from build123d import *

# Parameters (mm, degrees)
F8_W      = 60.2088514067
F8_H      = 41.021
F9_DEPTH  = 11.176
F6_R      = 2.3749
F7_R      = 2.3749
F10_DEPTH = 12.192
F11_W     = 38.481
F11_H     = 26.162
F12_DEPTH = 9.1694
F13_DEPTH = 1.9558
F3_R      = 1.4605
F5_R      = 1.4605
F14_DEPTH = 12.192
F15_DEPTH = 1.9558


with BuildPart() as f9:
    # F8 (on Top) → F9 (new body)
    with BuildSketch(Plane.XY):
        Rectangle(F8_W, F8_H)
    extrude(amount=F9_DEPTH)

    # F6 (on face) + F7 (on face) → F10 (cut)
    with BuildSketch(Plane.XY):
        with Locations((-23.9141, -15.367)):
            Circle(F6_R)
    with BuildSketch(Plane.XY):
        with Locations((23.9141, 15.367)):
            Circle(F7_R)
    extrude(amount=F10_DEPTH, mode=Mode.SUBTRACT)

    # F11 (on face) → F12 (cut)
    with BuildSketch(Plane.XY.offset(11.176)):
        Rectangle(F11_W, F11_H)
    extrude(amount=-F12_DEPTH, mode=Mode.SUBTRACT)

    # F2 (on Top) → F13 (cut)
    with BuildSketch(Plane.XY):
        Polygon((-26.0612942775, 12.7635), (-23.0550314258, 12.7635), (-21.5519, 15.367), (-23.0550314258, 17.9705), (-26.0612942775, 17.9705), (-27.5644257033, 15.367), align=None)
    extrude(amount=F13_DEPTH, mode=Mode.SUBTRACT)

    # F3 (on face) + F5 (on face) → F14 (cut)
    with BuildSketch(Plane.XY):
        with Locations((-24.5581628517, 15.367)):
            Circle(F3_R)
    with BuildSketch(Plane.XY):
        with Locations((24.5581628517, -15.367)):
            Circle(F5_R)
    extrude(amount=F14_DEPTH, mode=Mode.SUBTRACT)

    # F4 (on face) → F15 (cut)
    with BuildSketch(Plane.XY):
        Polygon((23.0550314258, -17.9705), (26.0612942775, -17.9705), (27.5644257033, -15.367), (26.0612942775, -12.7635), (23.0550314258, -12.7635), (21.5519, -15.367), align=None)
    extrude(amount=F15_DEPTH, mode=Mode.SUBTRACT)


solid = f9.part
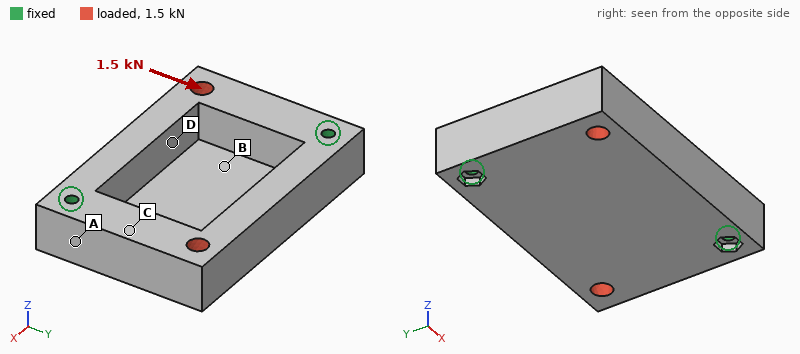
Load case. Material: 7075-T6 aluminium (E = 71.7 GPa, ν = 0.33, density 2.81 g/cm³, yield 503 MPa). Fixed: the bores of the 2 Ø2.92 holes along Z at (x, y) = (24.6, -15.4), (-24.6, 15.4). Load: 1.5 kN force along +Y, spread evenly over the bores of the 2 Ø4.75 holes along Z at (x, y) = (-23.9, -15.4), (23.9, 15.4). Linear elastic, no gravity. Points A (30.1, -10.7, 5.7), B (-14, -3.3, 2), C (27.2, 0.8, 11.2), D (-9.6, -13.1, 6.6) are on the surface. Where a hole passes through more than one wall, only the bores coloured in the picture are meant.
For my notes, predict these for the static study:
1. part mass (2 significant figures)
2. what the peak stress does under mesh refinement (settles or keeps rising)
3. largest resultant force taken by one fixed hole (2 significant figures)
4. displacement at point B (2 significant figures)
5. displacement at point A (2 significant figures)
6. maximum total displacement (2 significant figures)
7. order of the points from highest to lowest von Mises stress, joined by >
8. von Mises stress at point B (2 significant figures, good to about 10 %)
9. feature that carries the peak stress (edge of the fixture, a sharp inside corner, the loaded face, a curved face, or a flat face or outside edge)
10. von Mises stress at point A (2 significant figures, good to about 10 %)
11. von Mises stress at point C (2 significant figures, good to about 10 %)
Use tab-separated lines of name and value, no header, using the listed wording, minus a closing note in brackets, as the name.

part mass	50 g
what the peak stress does under mesh refinement	keeps rising
largest resultant force taken by one fixed hole	750 N
displacement at point B	1.8 µm
displacement at point A	0.65 µm
maximum total displacement	3.6 µm
order of the points from highest to lowest von Mises stress, joined by >	C > A > B > D
von Mises stress at point B	2.9 MPa
feature that carries the peak stress	edge of the fixture
von Mises stress at point A	4.9 MPa
von Mises stress at point C	6.7 MPa
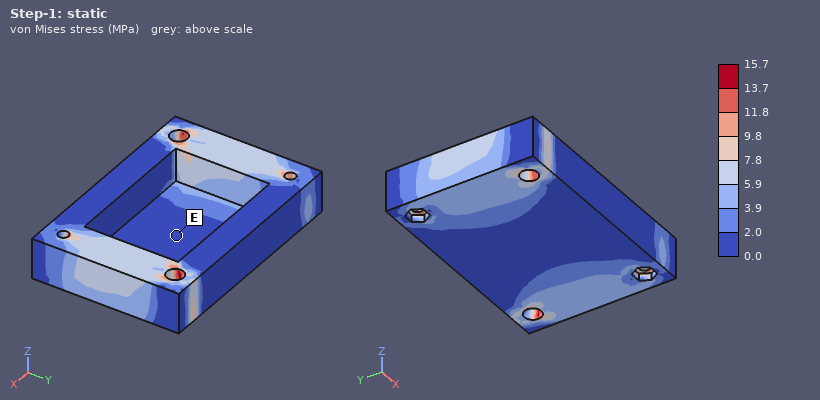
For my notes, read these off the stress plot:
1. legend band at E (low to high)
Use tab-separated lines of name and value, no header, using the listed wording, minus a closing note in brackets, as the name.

legend band at E	0.0 to 2.0 MPa
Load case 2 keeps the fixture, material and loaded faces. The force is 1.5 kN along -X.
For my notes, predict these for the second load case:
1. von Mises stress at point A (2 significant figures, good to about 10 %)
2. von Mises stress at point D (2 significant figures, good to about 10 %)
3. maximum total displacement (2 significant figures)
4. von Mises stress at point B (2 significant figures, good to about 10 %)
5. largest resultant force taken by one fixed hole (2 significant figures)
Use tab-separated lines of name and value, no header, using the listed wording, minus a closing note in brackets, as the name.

von Mises stress at point A	2.8 MPa
von Mises stress at point D	6.7 MPa
maximum total displacement	6.0 µm
von Mises stress at point B	2.3 MPa
largest resultant force taken by one fixed hole	750 N
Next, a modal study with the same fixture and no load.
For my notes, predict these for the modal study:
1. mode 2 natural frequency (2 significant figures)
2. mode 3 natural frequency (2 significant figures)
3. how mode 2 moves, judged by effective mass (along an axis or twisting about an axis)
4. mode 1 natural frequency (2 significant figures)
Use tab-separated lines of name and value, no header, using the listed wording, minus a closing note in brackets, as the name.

mode 2 natural frequency	7100 Hz
mode 3 natural frequency	13 kHz
how mode 2 moves, judged by effective mass	along Z
mode 1 natural frequency	5700 Hz
